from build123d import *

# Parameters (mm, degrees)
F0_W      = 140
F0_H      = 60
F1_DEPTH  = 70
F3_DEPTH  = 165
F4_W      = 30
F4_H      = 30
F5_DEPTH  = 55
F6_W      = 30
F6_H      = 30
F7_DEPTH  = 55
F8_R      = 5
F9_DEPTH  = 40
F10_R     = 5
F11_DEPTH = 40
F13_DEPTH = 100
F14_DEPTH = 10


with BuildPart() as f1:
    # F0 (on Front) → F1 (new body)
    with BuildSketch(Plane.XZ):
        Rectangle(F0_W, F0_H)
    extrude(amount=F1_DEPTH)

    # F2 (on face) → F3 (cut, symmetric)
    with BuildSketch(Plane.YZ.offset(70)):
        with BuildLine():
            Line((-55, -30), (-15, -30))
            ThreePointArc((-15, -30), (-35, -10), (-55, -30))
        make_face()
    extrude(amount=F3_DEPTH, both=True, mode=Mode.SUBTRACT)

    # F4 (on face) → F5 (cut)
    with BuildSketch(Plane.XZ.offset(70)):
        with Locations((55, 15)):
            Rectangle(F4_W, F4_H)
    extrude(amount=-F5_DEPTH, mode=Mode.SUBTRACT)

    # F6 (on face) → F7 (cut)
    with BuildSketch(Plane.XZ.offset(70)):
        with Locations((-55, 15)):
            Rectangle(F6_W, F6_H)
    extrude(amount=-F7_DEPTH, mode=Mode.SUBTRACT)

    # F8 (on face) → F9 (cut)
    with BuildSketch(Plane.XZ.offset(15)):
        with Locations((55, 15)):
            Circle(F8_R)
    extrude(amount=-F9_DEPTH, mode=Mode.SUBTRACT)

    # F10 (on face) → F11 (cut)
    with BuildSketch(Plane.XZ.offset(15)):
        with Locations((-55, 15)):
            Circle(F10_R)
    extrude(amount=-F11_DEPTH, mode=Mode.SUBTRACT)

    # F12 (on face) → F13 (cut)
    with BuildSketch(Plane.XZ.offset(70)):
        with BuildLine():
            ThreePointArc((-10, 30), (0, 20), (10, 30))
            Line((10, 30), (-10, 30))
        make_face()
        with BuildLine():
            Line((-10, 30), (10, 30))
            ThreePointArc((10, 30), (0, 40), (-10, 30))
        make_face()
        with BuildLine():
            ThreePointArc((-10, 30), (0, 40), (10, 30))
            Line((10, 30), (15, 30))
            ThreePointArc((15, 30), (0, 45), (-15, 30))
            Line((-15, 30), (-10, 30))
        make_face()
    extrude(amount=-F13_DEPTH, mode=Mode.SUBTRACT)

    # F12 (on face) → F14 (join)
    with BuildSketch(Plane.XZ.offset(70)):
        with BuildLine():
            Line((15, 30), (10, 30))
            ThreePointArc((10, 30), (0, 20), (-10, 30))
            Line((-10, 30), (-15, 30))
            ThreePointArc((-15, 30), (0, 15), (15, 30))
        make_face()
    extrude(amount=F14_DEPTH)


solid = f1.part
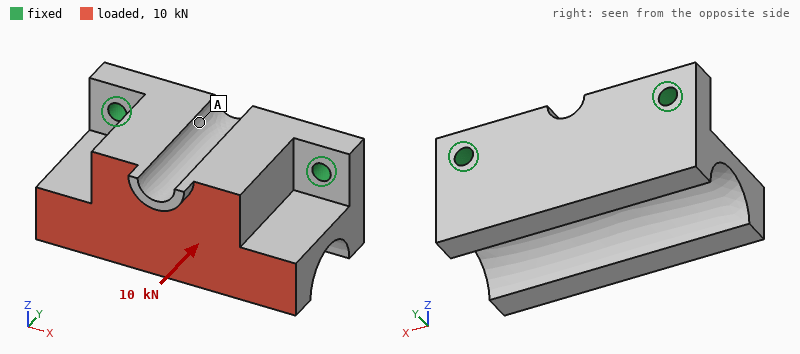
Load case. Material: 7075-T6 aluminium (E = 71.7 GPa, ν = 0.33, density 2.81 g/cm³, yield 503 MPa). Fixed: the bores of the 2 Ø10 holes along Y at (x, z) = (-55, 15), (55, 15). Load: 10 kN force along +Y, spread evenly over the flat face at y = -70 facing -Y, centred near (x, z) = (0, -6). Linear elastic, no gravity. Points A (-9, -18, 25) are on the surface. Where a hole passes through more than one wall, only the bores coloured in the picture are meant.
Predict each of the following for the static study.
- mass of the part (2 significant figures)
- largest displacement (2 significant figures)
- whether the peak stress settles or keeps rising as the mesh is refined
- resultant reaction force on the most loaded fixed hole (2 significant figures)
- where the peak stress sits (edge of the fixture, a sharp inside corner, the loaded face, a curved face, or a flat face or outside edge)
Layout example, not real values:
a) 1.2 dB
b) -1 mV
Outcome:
a) 1.1 kg
b) 98 µm
c) keeps rising
d) 5.1 kN
e) edge of the fixture
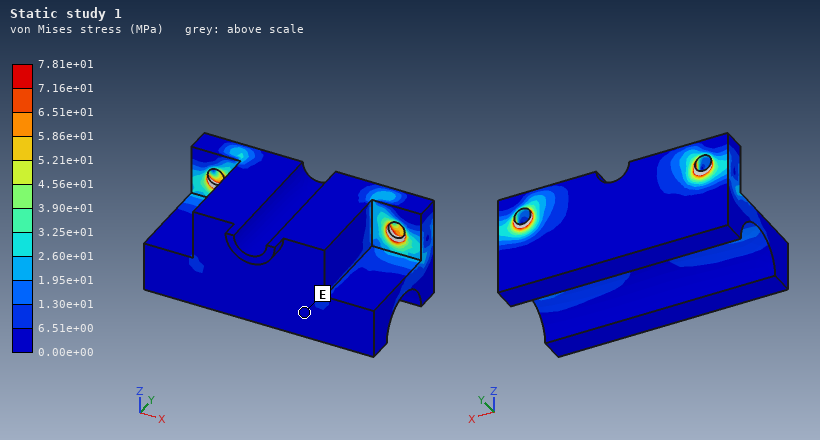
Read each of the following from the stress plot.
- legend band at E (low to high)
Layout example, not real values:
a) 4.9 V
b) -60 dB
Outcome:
a) 0.00e+00 to 6.51e+00 MPa
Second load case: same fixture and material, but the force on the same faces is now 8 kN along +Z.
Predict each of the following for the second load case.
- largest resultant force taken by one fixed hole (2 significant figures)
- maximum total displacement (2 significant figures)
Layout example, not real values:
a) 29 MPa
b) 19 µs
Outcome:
a) 4.7 kN
b) 0.29 mm
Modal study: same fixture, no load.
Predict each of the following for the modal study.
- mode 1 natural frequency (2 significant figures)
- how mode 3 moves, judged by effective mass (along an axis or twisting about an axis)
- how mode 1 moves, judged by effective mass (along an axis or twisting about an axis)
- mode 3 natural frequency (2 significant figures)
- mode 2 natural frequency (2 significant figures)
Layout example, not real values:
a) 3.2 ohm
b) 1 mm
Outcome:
a) 1400 Hz
b) along X
c) along Z
d) 4800 Hz
e) 4600 Hz
